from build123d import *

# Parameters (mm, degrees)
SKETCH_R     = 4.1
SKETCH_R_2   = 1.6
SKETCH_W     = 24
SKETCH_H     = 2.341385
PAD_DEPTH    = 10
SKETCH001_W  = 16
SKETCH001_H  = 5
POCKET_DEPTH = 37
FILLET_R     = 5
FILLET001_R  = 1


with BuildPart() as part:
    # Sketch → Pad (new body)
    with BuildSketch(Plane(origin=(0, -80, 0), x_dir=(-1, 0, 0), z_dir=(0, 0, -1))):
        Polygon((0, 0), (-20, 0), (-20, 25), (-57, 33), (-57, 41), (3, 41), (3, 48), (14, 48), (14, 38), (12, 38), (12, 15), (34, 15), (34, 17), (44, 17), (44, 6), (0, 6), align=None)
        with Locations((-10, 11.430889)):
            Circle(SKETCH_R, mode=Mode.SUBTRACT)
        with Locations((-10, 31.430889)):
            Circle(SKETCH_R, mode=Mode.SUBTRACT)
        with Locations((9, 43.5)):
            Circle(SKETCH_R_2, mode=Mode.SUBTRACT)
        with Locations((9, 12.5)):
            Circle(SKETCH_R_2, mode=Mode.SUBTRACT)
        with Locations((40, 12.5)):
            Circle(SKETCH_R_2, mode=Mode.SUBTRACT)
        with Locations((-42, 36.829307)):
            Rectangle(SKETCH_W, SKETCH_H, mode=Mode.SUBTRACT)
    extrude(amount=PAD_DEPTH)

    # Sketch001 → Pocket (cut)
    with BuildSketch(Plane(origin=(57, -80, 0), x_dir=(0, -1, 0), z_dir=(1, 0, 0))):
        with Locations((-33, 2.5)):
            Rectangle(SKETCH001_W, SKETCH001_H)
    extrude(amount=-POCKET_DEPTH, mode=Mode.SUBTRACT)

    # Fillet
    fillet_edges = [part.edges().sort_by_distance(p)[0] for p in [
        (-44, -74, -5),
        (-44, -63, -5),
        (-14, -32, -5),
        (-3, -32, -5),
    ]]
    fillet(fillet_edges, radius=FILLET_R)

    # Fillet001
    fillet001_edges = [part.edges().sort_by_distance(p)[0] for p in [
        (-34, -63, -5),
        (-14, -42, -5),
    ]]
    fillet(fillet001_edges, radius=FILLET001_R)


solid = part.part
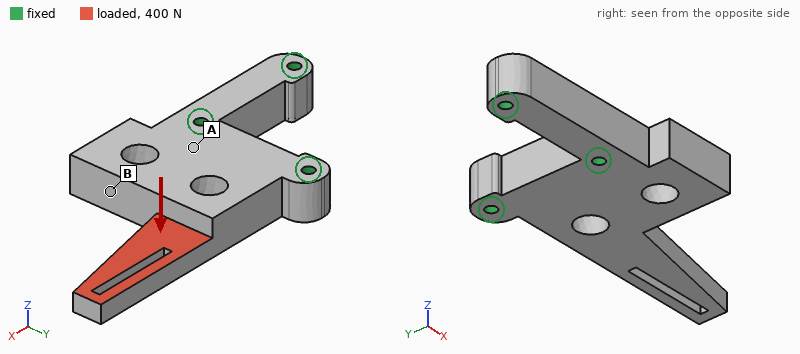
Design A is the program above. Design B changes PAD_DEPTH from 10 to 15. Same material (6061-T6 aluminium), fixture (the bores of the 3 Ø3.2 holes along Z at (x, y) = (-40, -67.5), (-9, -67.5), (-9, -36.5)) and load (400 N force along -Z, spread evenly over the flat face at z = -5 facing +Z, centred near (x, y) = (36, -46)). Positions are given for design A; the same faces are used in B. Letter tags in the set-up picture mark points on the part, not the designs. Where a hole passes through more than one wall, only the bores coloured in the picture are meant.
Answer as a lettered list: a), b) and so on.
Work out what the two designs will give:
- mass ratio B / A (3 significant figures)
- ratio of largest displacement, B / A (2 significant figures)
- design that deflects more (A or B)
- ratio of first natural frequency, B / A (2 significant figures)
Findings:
a) 1.56
b) 0.22
c) A
d) 1.4
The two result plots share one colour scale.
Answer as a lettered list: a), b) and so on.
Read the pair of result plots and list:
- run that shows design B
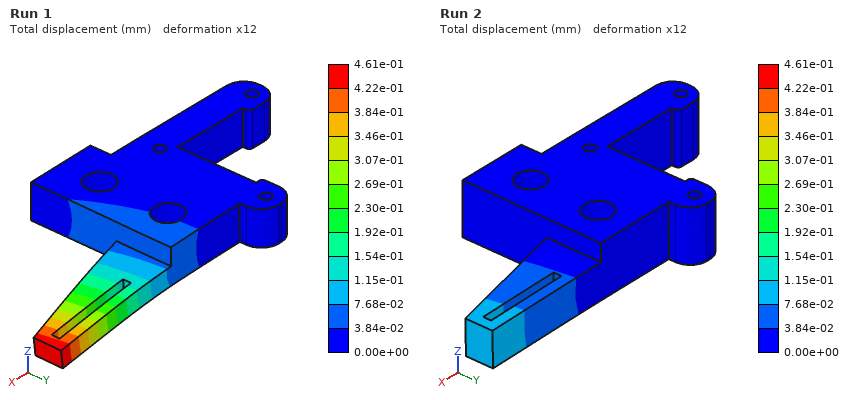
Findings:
a) Run 2
